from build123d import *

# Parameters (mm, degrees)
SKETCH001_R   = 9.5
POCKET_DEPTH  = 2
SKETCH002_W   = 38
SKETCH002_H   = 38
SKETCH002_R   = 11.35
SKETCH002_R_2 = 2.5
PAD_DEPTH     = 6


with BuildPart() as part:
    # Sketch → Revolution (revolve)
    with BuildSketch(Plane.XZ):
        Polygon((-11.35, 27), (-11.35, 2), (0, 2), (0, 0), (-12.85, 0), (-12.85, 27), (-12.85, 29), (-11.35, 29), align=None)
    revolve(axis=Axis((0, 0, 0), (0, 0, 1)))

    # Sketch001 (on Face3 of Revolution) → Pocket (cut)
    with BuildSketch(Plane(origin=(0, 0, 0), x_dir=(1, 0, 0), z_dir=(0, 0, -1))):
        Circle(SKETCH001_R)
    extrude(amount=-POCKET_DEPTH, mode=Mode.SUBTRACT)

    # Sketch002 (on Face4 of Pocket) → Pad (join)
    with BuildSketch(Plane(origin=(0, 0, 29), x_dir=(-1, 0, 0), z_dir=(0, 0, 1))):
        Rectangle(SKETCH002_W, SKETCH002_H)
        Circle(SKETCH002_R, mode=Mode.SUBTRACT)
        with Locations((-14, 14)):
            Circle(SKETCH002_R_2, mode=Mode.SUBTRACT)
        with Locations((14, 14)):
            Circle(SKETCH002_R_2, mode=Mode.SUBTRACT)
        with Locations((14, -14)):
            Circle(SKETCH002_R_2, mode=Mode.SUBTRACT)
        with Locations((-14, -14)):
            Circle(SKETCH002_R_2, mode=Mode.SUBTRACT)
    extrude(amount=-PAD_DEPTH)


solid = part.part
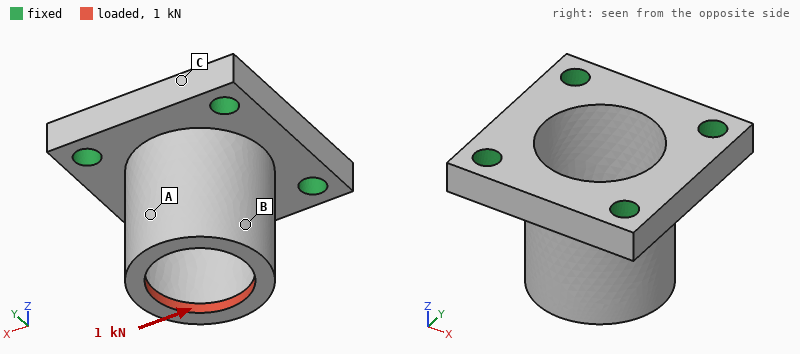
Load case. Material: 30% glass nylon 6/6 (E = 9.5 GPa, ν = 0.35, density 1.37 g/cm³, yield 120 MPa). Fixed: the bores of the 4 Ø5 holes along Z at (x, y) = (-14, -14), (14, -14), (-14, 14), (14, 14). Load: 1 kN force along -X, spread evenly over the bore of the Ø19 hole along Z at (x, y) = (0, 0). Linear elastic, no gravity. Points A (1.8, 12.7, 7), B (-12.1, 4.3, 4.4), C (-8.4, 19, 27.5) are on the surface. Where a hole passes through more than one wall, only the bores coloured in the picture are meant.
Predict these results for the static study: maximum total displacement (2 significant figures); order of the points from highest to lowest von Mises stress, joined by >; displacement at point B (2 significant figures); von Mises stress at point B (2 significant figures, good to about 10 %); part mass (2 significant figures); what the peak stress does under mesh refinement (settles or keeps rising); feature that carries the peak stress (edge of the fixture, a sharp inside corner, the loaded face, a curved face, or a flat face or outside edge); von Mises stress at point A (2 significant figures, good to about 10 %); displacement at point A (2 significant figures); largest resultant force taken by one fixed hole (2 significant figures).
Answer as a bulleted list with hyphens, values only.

- 0.29 mm
- A > B > C
- 0.22 mm
- 17 MPa
- 12 g
- keeps rising
- edge of the fixture
- 28 MPa
- 0.17 mm
- 590 N
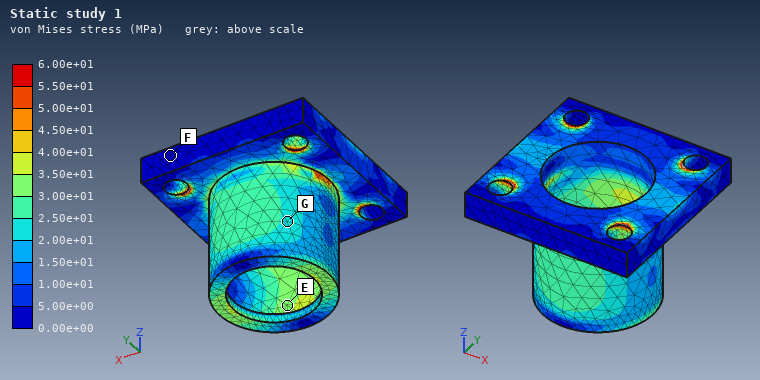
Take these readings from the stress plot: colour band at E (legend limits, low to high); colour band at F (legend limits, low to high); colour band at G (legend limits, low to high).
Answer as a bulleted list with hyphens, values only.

- 3.00e+01 to 3.50e+01 MPa
- 0.00e+00 to 5.00e+00 MPa
- 2.00e+01 to 2.50e+01 MPa
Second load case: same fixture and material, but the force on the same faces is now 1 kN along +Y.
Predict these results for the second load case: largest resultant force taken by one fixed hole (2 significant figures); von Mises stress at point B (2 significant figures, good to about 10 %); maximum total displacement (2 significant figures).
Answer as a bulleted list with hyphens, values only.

- 590 N
- 24 MPa
- 0.29 mm
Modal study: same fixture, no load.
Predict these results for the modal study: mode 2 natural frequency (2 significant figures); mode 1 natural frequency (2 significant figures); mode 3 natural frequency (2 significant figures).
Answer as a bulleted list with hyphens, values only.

- 7400 Hz
- 7400 Hz
- 7500 Hz
